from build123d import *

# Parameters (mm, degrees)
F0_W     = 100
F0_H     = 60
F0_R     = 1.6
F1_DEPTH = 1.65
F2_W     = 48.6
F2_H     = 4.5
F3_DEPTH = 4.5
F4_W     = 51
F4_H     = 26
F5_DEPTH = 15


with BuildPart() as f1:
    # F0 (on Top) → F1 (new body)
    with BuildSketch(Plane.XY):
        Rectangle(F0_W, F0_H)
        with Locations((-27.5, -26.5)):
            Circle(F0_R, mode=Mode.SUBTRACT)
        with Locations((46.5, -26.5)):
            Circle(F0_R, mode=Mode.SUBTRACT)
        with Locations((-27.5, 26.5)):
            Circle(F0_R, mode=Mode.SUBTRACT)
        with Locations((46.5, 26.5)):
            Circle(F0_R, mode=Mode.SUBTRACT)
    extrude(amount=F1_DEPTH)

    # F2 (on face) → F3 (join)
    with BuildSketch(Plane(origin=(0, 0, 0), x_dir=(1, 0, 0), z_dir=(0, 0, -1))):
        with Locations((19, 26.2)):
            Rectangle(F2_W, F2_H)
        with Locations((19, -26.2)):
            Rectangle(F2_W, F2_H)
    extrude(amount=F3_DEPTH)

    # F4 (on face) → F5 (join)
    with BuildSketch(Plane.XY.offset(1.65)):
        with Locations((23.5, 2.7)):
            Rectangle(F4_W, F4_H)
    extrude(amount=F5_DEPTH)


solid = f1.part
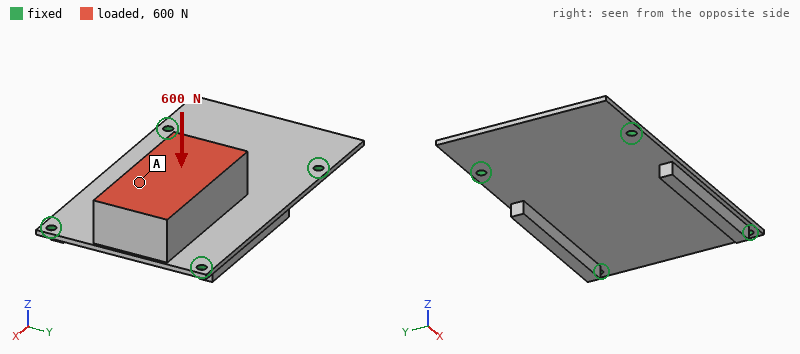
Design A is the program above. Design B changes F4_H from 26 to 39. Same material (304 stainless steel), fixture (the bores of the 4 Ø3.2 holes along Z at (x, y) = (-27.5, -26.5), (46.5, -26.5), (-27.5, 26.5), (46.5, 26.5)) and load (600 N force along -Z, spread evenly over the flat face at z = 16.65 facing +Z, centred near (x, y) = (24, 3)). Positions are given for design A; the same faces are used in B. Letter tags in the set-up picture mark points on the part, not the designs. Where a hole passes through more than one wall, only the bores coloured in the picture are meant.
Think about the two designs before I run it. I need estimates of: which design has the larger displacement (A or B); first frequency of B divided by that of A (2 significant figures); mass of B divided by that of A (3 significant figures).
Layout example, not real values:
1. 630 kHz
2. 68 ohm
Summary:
1. A
2. 0.95
3. 1.31
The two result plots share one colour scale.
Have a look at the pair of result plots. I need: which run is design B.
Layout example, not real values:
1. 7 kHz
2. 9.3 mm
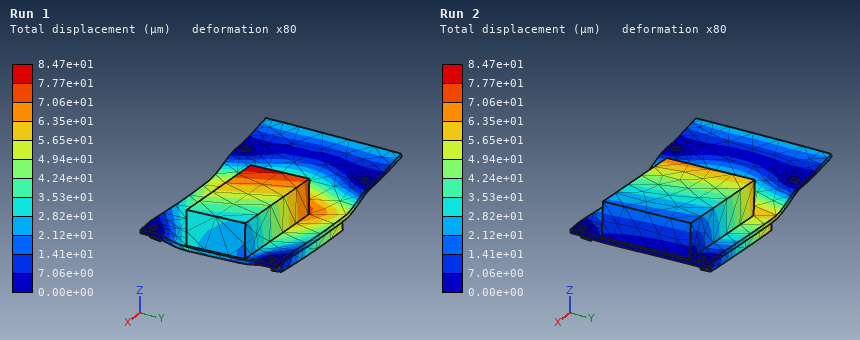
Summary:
1. Run 2
